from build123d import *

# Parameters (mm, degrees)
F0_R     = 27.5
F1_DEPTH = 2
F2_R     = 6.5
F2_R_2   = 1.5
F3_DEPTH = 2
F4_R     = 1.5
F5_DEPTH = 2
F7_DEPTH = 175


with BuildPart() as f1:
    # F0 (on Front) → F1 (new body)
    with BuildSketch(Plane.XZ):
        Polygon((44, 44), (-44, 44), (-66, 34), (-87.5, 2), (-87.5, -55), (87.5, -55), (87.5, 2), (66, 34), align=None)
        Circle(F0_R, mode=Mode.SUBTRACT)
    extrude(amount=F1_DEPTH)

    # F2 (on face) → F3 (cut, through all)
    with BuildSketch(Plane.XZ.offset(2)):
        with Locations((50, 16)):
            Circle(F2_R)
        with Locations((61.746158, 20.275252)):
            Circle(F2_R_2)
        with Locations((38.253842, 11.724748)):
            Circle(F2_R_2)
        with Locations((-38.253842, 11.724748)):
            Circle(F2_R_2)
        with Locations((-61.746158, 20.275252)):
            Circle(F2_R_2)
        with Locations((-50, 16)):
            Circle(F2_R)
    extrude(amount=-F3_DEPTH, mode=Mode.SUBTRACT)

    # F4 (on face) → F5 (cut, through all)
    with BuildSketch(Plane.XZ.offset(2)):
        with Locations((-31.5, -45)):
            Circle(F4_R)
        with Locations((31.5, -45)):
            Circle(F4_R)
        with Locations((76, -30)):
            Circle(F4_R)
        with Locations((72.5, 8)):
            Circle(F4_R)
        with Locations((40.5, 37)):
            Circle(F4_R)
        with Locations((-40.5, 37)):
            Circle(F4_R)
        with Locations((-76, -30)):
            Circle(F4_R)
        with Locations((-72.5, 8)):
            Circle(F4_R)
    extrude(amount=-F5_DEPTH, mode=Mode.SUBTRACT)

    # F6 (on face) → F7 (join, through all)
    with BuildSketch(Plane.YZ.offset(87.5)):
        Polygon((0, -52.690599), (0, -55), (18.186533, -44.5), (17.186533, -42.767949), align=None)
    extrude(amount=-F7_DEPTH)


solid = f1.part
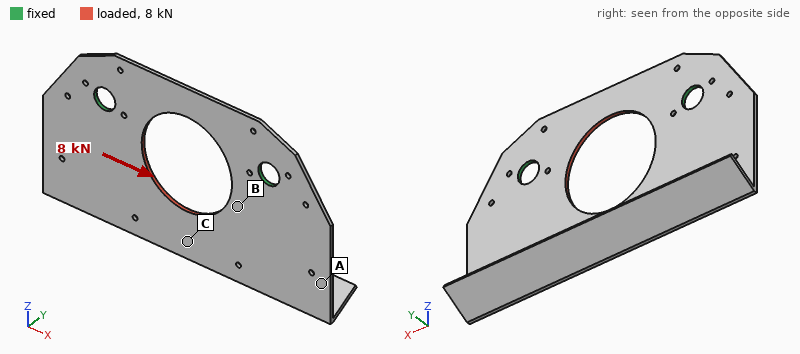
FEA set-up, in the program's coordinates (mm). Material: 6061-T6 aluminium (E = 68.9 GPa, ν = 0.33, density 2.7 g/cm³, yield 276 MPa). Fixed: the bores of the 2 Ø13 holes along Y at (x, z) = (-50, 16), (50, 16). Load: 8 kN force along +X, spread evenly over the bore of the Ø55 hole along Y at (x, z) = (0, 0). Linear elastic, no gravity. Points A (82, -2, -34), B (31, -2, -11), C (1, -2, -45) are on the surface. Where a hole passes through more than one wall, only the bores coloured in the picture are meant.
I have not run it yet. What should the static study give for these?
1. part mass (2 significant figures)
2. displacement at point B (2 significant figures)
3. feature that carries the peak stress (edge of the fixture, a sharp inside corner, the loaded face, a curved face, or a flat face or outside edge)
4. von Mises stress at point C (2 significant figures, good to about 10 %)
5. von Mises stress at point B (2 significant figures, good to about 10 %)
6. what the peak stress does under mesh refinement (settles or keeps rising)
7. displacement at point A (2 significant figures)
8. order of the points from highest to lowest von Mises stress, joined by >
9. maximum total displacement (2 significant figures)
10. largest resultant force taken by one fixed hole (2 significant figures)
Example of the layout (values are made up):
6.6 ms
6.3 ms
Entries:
91 g
51 µm
edge of the fixture
30 MPa
47 MPa
keeps rising
70 µm
B > C > A
90 µm
4.1 kN
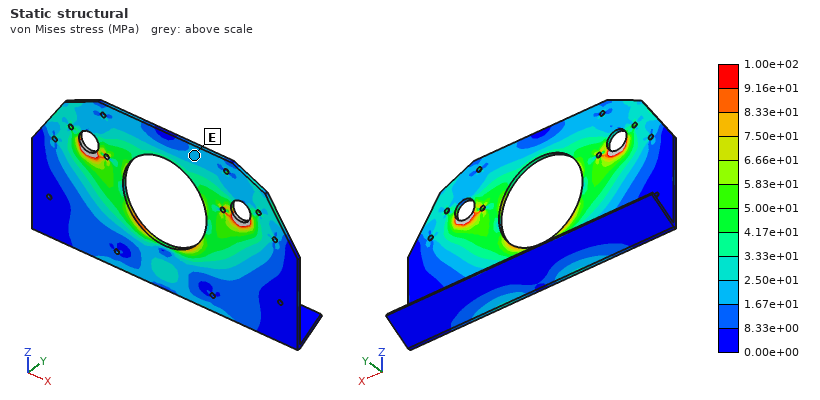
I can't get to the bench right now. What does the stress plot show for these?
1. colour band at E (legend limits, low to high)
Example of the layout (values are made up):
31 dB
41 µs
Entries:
1.67e+01 to 2.50e+01 MPa
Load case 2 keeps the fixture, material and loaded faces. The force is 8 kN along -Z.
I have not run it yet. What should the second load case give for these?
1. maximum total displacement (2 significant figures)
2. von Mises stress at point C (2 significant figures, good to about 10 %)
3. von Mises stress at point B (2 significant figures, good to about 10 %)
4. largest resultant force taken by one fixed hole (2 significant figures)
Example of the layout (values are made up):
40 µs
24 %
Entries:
71 µm
29 MPa
47 MPa
4.0 kN
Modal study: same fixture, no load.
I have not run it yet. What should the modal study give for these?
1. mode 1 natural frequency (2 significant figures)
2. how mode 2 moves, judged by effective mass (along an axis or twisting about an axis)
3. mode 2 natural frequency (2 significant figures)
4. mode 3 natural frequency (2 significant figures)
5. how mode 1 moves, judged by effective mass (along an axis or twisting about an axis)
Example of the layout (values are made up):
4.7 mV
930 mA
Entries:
210 Hz
twisting about Z
330 Hz
1200 Hz
along Y
